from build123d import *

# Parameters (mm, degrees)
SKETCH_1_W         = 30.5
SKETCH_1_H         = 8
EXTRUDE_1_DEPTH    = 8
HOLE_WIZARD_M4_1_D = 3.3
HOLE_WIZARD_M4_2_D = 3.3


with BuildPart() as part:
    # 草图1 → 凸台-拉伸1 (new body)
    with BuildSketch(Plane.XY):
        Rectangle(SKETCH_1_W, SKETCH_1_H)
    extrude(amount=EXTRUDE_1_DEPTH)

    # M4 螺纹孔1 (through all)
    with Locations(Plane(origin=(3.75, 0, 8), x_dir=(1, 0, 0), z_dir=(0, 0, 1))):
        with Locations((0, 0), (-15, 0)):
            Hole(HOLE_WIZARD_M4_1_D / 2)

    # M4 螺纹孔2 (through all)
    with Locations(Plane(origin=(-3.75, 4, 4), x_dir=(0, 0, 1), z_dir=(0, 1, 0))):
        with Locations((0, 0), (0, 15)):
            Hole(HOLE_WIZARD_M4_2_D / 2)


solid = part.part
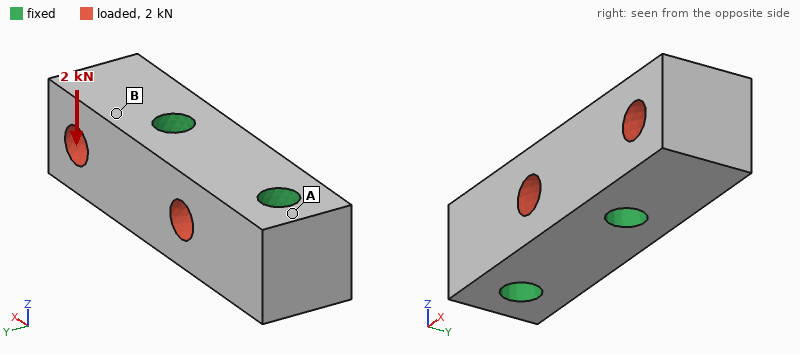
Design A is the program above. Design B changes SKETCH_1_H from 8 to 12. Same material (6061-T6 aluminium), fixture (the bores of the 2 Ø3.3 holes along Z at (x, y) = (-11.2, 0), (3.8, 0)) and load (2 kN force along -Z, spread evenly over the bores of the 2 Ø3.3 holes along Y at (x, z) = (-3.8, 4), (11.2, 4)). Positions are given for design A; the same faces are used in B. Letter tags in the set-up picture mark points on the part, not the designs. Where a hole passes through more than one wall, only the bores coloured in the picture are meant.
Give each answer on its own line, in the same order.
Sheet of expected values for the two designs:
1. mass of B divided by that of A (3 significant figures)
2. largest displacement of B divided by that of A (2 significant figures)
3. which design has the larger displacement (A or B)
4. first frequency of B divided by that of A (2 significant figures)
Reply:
1.54
0.76
A
1.0
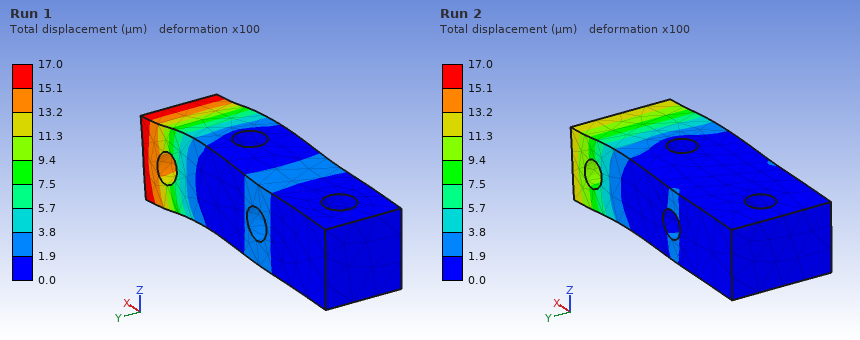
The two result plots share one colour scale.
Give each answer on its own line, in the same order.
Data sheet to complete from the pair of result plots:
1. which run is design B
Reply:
Run 2
